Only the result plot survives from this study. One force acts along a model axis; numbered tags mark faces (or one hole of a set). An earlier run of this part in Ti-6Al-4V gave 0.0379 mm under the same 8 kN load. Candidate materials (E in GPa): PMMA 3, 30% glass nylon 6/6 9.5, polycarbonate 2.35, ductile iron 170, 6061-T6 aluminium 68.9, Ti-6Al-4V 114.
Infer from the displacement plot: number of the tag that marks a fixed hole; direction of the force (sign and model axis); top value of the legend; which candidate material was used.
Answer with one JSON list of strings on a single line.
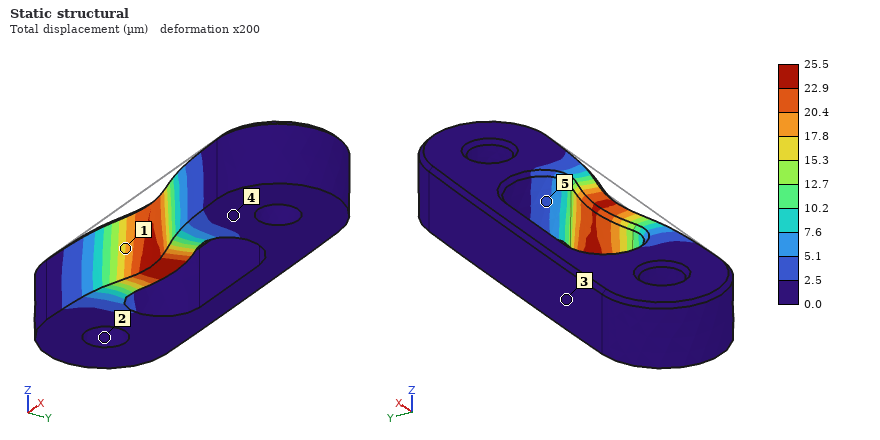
["2", "+Y", "25.5 µm", "ductile iron"]
